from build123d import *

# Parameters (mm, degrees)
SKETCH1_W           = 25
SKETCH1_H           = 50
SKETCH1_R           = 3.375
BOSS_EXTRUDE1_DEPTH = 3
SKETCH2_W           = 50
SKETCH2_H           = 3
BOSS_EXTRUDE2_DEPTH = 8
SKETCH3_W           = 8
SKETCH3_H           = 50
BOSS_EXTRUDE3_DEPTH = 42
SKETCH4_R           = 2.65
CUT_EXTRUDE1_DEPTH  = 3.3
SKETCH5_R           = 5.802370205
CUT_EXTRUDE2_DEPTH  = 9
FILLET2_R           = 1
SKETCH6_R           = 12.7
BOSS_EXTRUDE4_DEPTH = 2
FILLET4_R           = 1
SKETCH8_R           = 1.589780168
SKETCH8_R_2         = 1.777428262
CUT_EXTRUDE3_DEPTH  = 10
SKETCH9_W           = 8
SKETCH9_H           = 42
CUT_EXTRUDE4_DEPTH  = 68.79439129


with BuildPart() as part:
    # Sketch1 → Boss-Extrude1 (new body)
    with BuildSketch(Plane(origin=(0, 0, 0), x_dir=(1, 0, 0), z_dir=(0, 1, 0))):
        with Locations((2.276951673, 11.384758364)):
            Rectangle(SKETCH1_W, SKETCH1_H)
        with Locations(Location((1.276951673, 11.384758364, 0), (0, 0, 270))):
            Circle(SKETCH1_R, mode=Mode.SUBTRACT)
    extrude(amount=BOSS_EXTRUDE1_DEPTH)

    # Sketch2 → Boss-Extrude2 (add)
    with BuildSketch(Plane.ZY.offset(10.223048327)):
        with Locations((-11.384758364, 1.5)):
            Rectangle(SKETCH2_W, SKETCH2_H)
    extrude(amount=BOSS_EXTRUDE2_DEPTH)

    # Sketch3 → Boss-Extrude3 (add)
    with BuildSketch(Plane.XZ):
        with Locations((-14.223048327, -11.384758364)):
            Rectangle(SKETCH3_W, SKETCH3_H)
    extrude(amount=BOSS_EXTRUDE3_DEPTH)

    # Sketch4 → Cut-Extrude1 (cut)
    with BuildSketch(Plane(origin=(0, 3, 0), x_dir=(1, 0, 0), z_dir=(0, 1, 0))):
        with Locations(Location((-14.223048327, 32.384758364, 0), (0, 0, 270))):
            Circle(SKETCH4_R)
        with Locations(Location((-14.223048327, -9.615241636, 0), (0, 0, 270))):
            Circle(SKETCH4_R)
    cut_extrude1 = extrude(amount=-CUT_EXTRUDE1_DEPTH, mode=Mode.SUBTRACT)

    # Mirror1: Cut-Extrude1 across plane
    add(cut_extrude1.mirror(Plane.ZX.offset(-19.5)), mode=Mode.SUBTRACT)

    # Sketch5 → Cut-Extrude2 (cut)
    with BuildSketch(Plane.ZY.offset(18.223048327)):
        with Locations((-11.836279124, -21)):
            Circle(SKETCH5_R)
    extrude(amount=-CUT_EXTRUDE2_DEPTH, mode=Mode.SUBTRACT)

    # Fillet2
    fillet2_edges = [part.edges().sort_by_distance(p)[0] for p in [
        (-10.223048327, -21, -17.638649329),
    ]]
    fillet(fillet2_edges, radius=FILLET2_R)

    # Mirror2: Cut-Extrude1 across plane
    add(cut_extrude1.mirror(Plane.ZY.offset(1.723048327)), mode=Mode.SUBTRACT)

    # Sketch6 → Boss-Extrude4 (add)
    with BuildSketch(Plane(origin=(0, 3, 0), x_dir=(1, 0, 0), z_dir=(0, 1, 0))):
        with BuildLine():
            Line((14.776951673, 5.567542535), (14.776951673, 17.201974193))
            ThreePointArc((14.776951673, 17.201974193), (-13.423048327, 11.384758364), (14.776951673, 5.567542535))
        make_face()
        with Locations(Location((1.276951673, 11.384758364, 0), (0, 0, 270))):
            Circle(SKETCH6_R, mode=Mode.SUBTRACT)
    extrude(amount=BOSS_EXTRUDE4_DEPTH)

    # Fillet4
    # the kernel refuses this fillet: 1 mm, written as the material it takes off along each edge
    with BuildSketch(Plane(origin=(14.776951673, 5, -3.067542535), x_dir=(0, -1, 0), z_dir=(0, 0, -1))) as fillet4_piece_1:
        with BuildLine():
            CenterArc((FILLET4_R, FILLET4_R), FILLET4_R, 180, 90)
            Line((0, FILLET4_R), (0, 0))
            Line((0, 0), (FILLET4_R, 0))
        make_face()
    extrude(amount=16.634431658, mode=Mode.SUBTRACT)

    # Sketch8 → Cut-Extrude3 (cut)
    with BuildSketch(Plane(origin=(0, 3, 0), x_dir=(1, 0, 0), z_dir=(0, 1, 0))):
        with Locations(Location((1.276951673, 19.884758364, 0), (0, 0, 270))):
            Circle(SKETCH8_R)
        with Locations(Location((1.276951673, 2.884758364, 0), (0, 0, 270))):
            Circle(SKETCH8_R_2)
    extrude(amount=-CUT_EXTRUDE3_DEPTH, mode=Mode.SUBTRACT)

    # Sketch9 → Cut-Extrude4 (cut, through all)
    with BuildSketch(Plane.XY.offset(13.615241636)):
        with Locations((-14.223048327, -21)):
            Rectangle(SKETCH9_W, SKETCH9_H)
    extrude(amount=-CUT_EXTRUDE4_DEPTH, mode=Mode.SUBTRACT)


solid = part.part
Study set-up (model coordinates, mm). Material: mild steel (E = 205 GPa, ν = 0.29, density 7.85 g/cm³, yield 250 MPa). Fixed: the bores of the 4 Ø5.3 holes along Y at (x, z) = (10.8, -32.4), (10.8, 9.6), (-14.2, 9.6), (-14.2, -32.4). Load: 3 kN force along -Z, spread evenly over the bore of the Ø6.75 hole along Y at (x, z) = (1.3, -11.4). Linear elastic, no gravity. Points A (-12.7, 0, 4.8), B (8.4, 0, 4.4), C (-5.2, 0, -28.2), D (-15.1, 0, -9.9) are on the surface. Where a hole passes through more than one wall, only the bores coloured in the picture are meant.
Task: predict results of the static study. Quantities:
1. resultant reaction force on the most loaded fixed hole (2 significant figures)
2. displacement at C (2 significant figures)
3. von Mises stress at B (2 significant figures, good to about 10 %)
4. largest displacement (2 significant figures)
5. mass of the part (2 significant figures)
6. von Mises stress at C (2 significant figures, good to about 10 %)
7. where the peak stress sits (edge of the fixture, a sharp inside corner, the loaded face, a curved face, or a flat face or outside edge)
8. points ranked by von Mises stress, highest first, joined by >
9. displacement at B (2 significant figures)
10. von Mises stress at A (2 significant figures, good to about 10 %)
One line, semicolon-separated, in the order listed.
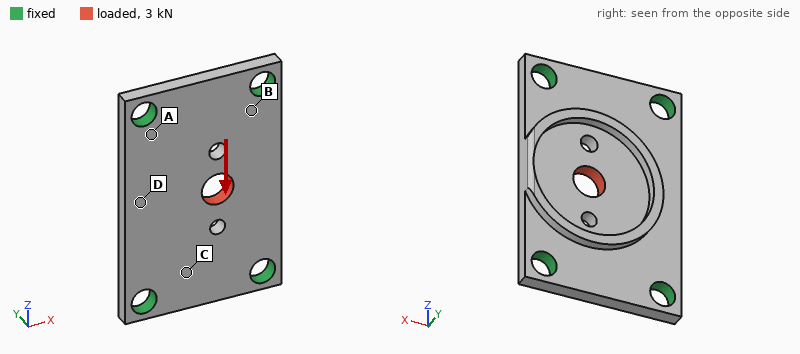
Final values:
890 N; 1.00 µm; 33 MPa; 3.4 µm; 38 g; 14 MPa; a curved face; B > A > C > D; 0.55 µm; 25 MPa
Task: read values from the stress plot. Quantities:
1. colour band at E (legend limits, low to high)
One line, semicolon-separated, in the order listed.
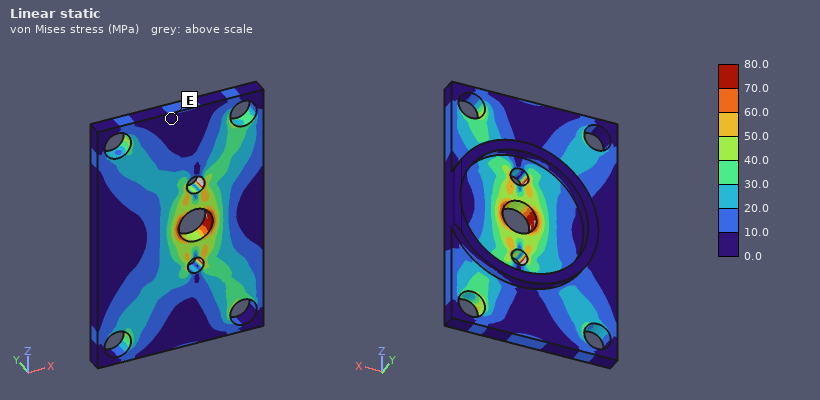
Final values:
0.0 to 10.0 MPa
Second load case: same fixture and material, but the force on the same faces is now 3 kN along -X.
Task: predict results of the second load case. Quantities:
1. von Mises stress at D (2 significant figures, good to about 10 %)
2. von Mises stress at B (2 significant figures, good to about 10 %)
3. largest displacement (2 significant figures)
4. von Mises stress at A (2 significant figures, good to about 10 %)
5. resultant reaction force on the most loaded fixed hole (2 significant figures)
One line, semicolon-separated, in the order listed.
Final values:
15 MPa; 32 MPa; 5.9 µm; 36 MPa; 970 N
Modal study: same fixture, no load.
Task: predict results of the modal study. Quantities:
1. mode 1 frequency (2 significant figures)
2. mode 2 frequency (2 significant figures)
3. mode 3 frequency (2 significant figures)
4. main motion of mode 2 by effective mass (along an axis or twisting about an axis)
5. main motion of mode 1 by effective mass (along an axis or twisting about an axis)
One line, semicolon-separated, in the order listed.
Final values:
9600 Hz; 13 kHz; 22 kHz; twisting about Z; along Y
